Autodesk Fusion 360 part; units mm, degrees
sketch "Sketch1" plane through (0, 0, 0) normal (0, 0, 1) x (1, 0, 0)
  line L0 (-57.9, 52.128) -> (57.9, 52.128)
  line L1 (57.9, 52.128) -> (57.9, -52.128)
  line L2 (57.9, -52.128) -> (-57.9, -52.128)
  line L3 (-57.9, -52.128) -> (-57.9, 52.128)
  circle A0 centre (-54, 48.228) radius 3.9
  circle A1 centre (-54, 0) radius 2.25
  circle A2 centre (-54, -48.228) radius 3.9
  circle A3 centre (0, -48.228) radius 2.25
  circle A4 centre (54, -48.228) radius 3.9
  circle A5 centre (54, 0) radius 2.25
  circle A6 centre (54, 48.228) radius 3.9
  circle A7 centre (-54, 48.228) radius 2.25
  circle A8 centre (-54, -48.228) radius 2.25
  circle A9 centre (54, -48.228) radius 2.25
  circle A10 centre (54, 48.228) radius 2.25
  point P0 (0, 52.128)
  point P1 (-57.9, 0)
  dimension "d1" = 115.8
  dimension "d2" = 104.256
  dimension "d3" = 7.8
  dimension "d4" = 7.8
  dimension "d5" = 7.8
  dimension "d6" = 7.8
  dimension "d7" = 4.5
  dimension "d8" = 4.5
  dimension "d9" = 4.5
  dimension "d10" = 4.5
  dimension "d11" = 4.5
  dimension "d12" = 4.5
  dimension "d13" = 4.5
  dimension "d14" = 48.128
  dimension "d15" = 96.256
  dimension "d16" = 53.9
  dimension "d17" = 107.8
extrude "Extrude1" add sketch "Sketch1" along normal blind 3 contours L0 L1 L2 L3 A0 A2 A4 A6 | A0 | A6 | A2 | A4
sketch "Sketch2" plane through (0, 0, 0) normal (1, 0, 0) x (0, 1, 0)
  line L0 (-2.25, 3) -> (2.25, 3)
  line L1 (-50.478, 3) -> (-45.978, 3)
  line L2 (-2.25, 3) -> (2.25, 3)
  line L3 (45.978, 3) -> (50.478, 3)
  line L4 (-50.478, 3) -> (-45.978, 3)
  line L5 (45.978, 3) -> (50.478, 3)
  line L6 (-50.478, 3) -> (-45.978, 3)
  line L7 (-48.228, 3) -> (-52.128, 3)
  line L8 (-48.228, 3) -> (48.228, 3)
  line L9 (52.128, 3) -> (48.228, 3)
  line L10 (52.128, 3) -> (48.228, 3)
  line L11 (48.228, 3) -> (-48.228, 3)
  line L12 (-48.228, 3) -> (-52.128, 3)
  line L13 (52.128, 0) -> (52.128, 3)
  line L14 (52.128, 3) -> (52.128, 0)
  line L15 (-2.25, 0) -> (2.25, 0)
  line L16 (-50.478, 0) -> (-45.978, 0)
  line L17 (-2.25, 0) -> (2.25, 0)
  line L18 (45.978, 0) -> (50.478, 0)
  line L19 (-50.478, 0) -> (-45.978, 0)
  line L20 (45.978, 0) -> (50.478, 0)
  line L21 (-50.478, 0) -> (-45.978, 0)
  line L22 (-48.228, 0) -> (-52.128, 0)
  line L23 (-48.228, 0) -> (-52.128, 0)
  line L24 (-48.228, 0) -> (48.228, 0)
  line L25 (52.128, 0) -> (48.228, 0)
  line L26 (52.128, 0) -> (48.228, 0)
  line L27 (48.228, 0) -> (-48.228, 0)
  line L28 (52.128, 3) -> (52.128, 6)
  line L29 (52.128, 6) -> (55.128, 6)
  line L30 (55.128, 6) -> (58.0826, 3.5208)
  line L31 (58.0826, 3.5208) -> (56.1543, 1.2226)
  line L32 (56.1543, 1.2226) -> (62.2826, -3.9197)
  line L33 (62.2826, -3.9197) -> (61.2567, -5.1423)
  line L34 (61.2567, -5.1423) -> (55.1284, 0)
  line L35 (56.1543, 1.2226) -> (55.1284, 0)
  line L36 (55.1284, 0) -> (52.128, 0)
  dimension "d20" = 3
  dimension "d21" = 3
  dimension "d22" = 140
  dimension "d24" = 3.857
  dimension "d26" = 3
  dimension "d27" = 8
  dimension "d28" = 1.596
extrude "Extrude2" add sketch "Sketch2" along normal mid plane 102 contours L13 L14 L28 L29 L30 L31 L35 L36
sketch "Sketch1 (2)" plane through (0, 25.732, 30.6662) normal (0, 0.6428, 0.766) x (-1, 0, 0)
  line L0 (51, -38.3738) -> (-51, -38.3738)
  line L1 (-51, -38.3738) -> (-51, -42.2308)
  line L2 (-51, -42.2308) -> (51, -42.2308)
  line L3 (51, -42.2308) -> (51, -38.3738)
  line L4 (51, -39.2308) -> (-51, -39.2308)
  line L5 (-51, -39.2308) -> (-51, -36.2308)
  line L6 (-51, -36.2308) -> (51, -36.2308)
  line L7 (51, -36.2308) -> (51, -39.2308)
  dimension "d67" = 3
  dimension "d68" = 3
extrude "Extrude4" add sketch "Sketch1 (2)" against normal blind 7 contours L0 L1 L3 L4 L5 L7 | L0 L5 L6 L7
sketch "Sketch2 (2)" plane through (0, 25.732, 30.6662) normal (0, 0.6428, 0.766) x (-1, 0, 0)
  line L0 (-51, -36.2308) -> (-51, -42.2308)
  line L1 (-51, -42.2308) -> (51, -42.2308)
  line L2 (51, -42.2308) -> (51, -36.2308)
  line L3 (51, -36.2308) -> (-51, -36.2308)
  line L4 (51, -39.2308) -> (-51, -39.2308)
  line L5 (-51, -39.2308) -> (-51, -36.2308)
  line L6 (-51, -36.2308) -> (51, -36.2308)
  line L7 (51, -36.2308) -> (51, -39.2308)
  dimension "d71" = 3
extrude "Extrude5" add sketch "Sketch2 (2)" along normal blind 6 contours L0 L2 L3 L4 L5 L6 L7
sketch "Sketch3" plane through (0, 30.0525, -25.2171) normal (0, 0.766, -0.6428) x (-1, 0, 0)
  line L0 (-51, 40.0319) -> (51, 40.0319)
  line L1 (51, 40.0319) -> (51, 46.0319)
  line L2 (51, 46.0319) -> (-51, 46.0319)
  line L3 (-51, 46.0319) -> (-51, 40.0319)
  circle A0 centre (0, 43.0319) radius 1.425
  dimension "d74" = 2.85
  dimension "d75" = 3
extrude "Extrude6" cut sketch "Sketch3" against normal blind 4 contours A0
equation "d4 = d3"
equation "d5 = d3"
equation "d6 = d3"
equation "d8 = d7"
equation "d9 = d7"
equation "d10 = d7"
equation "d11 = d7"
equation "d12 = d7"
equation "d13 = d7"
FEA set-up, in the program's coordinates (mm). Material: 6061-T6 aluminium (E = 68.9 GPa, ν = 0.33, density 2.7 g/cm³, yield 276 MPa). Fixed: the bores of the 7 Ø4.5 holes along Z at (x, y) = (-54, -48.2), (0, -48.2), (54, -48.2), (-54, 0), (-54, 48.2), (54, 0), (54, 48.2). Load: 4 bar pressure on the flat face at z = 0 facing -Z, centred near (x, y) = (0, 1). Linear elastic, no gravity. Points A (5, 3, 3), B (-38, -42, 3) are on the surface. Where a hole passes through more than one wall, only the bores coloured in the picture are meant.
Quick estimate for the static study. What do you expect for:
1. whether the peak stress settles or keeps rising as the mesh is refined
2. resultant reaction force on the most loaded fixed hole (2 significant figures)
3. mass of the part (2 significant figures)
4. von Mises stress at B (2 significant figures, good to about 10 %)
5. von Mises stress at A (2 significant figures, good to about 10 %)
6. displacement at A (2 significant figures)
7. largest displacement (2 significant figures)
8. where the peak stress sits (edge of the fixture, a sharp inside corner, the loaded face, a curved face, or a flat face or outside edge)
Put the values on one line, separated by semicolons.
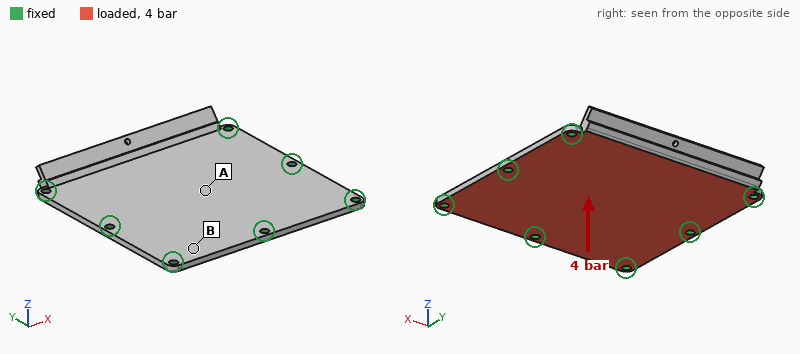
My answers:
keeps rising; 1.3 kN; 110 g; 35 MPa; 82 MPa; 0.58 mm; 0.60 mm; edge of the fixture
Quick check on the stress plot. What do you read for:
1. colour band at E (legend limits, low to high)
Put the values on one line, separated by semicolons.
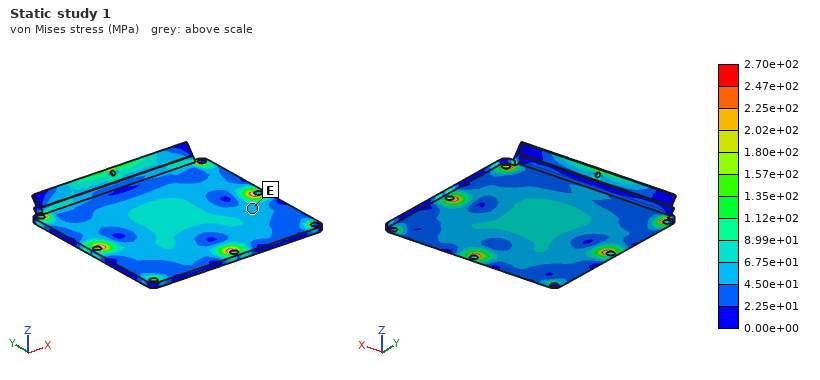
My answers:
4.50e+01 to 6.75e+01 MPa
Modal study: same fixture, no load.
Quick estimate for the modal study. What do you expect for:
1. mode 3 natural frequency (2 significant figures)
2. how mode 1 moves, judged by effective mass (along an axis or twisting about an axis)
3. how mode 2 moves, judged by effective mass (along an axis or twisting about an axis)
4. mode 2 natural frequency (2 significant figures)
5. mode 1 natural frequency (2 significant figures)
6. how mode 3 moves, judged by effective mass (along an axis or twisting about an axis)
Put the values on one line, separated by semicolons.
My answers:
3700 Hz; along Z; twisting about X; 2700 Hz; 1800 Hz; twisting about Y
